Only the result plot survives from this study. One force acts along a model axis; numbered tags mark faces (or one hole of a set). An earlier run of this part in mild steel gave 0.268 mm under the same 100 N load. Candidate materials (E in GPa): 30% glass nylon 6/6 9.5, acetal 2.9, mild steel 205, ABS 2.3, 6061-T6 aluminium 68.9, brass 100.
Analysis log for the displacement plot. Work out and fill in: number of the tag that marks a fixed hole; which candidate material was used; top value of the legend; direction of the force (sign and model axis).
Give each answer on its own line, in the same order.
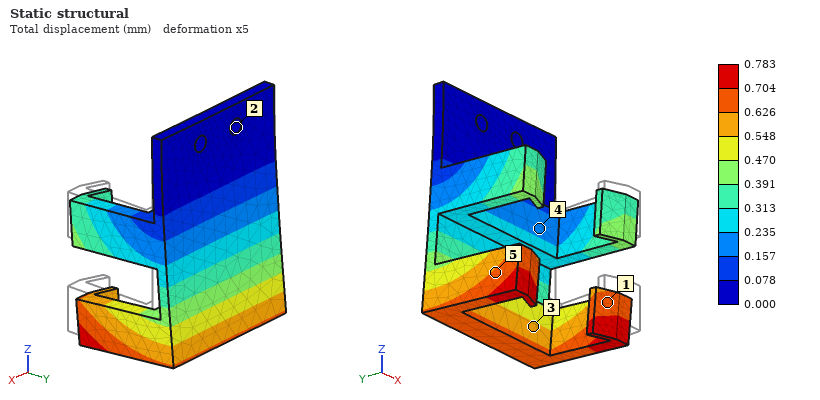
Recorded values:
2
6061-T6 aluminium
0.783 mm
+Y
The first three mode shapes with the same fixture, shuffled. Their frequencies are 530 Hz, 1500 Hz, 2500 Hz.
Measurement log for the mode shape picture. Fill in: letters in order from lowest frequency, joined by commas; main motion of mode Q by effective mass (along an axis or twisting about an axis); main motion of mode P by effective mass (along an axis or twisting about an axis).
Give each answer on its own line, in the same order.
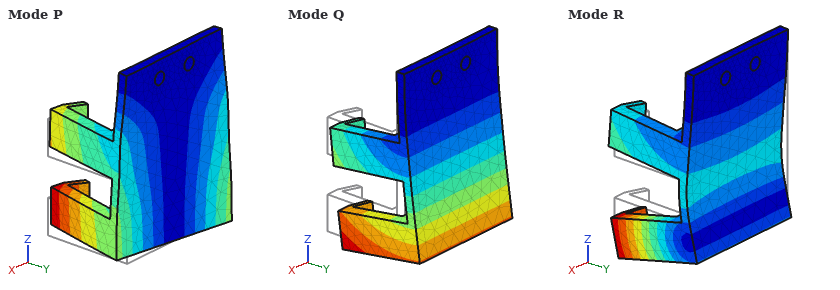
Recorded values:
Q, P, R
along Y
along X
